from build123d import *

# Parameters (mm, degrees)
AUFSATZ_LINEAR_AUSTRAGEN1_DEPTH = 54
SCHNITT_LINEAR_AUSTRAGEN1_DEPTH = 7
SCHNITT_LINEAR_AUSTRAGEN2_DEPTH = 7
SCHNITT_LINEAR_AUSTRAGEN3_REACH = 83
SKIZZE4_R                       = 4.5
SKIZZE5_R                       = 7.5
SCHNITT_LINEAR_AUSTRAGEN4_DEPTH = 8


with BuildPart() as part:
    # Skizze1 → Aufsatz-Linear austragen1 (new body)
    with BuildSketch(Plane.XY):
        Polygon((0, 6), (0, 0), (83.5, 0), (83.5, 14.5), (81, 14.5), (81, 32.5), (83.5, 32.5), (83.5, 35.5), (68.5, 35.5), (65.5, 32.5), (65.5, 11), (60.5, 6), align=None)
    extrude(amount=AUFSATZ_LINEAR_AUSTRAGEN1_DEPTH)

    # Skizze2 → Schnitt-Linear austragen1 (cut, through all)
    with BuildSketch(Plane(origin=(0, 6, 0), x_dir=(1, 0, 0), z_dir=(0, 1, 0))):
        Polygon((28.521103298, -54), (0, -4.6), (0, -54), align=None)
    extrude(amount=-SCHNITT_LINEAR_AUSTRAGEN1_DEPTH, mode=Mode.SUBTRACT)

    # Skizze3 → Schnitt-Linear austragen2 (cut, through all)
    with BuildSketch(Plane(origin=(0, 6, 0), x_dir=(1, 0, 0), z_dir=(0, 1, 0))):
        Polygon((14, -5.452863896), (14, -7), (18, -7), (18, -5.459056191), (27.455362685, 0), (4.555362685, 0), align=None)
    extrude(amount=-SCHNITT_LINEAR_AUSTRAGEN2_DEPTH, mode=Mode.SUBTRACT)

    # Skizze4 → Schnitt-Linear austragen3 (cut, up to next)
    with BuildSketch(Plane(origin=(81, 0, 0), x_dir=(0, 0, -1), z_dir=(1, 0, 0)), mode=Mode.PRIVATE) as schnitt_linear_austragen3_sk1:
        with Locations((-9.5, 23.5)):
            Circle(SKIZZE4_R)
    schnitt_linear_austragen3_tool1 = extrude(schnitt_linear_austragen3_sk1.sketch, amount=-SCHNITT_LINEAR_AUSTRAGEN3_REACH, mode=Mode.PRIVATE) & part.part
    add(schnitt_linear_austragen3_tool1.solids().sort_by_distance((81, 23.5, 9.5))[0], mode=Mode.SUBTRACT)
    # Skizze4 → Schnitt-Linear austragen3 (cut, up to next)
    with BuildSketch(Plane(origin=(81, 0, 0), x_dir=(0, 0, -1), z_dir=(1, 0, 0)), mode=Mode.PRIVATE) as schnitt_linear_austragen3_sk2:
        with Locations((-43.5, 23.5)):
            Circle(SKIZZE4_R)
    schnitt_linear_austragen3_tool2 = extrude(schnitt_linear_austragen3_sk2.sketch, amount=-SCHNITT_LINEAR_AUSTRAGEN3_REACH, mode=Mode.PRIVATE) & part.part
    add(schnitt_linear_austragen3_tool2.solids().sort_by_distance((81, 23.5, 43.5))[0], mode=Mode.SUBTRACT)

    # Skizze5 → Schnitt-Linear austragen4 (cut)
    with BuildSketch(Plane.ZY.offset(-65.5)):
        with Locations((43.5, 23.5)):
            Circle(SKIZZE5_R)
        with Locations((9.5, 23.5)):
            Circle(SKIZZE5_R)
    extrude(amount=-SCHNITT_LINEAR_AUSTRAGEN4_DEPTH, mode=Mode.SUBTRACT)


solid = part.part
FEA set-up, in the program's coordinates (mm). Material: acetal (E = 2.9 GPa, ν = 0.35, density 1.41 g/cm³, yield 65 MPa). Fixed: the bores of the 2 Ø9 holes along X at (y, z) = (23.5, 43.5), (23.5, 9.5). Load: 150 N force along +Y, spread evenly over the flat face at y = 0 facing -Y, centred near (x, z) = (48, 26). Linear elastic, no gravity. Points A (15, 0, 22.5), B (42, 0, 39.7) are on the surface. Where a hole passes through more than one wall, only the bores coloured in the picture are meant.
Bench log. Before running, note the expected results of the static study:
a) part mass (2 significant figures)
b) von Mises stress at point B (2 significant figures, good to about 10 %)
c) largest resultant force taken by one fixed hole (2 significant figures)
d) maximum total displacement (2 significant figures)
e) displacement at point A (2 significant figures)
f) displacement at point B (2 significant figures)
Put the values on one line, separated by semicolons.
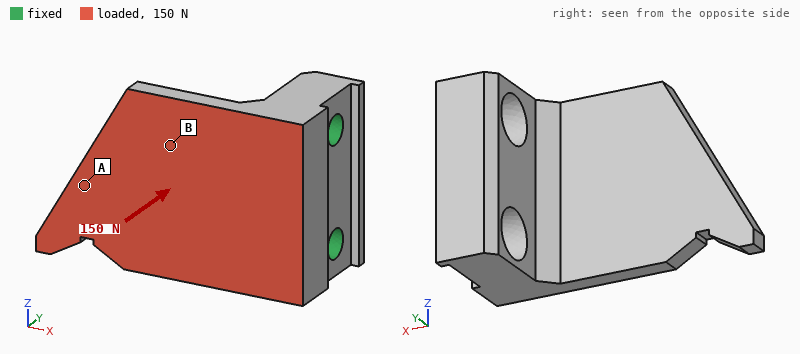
64 g; 2.6 MPa; 81 N; 1.2 mm; 0.82 mm; 0.29 mm
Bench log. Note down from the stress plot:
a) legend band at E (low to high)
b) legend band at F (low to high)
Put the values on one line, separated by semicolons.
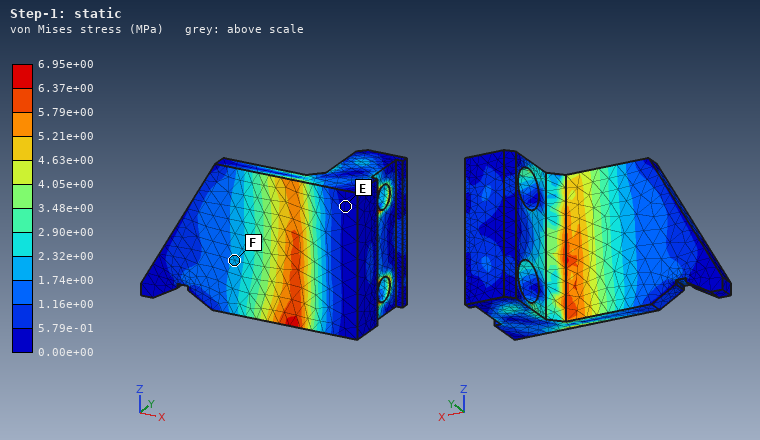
0.00e+00 to 5.79e-01 MPa; 1.74e+00 to 2.32e+00 MPa
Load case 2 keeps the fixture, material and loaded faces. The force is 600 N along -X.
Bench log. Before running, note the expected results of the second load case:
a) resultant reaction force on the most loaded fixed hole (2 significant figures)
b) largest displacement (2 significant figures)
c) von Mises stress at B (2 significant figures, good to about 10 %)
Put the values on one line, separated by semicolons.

320 N; 1.3 mm; 2.6 MPa
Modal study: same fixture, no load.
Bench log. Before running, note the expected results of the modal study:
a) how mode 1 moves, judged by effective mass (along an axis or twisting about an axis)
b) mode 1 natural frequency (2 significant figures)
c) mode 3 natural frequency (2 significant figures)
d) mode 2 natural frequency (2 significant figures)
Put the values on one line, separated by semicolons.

along Y; 450 Hz; 1500 Hz; 1200 Hz
